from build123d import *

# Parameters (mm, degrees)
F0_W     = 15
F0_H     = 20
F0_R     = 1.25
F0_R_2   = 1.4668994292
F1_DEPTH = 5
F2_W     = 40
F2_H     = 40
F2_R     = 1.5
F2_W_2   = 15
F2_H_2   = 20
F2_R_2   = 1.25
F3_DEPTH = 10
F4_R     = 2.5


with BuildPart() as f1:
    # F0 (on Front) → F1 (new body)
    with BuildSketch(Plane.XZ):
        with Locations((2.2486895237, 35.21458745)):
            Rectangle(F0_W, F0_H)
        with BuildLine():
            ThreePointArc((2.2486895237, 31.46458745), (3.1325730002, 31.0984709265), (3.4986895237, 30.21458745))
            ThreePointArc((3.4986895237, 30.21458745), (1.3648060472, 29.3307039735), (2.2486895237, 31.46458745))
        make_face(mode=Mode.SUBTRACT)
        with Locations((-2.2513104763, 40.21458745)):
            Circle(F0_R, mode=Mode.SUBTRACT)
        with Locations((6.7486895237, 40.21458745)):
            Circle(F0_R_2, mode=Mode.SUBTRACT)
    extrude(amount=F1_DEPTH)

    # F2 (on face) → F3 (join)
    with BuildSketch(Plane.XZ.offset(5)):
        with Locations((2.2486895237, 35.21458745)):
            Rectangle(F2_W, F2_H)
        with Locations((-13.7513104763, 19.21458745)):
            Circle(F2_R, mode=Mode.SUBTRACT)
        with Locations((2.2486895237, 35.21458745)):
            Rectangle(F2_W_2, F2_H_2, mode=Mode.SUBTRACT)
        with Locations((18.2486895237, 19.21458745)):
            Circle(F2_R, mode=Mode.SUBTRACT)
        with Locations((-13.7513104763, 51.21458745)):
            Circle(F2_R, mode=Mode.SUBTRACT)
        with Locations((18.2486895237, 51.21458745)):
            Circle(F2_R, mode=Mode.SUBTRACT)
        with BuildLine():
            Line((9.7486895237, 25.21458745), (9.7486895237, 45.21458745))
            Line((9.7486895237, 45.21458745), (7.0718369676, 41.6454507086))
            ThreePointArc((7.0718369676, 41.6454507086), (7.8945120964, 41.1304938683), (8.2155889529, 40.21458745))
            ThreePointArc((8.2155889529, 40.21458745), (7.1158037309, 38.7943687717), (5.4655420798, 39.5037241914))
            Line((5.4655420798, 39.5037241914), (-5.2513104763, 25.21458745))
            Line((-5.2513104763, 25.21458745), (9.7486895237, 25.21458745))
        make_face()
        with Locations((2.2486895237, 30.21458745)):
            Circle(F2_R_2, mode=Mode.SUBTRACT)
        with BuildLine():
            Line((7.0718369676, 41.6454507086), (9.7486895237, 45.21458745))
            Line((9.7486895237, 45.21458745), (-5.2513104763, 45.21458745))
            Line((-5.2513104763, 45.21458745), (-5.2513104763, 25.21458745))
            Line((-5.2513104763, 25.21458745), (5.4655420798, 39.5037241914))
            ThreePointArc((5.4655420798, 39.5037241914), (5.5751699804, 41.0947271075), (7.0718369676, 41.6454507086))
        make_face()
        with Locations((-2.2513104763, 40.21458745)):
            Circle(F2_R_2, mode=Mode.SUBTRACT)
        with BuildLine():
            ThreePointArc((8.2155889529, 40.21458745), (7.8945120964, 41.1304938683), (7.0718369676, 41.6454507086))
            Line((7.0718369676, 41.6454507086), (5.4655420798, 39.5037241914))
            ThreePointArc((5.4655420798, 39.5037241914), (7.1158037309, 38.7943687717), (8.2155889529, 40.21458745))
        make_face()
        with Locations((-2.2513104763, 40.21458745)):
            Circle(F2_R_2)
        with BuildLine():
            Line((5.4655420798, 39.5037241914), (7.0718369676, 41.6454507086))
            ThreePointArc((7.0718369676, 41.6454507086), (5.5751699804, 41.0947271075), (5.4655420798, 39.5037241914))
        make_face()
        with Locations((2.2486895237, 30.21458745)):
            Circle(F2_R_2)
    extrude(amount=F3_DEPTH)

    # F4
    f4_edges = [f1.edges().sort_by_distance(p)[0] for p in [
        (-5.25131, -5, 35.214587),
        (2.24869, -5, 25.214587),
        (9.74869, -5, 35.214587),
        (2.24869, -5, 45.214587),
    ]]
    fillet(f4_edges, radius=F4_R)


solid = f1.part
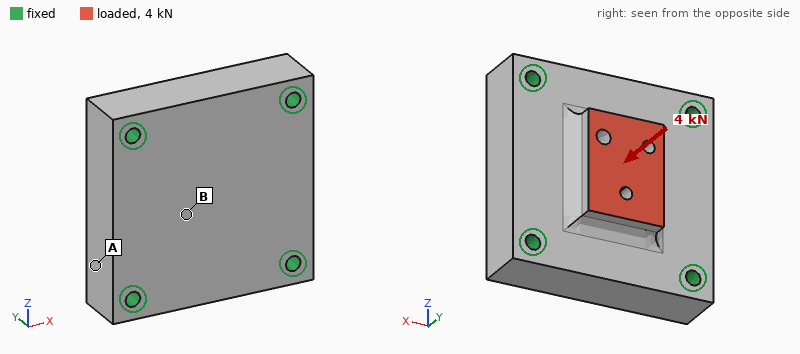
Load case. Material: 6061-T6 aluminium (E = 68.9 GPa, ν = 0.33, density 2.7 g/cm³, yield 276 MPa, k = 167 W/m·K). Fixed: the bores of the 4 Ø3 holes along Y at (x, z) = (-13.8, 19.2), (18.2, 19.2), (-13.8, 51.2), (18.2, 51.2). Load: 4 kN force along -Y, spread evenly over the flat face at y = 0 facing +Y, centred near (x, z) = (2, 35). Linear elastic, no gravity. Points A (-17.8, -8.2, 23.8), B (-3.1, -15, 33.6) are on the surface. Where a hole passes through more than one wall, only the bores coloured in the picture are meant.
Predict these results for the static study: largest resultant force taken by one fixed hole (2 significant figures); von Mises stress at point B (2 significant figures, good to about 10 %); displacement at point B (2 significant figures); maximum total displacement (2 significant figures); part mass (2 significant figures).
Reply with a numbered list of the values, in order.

1. 1.0 kN
2. 17 MPa
3. 7.8 µm
4. 9.3 µm
5. 47 g
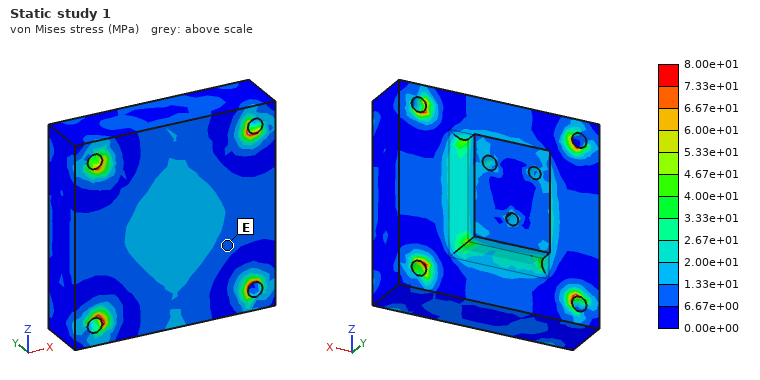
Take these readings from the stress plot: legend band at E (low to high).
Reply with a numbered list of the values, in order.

1. 6.67e+00 to 1.33e+01 MPa
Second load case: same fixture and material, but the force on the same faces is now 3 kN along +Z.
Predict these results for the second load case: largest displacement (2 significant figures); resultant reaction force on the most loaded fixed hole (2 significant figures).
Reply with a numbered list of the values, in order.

1. 9.1 µm
2. 980 N
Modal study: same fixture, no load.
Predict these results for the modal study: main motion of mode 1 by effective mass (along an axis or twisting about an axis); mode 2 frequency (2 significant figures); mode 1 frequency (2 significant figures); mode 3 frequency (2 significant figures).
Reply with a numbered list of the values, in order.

1. along Y
2. 33 kHz
3. 23 kHz
4. 34 kHz
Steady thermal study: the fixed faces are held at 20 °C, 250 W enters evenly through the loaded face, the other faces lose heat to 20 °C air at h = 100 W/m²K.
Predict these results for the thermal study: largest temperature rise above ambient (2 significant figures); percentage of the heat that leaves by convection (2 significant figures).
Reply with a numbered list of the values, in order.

1. 73 K
2. 3.9 %
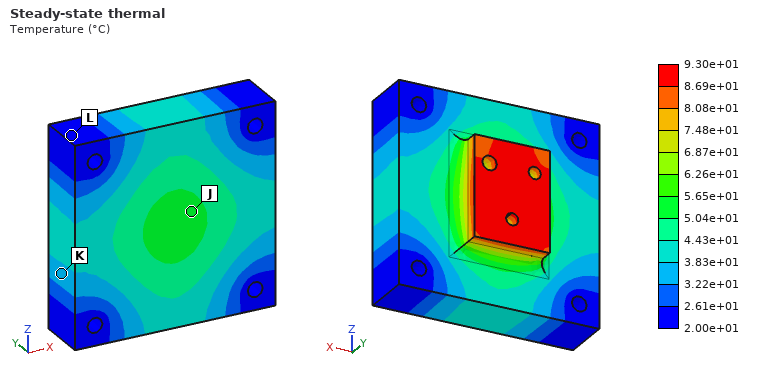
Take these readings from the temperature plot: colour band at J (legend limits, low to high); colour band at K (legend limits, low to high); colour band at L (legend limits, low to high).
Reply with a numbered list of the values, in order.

1. 5.04e+01 to 5.65e+01 °C
2. 3.22e+01 to 3.83e+01 °C
3. 2.00e+01 to 2.61e+01 °C
